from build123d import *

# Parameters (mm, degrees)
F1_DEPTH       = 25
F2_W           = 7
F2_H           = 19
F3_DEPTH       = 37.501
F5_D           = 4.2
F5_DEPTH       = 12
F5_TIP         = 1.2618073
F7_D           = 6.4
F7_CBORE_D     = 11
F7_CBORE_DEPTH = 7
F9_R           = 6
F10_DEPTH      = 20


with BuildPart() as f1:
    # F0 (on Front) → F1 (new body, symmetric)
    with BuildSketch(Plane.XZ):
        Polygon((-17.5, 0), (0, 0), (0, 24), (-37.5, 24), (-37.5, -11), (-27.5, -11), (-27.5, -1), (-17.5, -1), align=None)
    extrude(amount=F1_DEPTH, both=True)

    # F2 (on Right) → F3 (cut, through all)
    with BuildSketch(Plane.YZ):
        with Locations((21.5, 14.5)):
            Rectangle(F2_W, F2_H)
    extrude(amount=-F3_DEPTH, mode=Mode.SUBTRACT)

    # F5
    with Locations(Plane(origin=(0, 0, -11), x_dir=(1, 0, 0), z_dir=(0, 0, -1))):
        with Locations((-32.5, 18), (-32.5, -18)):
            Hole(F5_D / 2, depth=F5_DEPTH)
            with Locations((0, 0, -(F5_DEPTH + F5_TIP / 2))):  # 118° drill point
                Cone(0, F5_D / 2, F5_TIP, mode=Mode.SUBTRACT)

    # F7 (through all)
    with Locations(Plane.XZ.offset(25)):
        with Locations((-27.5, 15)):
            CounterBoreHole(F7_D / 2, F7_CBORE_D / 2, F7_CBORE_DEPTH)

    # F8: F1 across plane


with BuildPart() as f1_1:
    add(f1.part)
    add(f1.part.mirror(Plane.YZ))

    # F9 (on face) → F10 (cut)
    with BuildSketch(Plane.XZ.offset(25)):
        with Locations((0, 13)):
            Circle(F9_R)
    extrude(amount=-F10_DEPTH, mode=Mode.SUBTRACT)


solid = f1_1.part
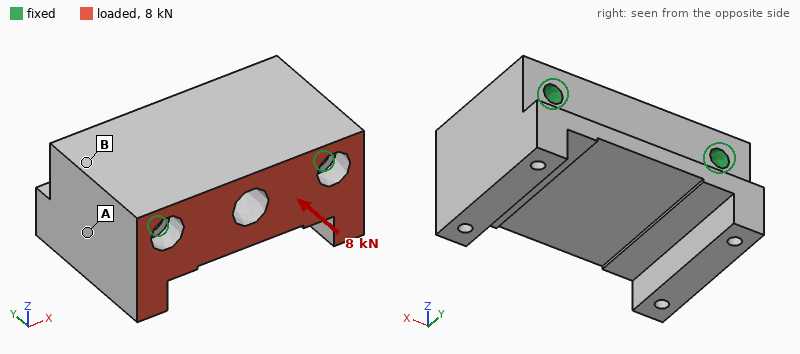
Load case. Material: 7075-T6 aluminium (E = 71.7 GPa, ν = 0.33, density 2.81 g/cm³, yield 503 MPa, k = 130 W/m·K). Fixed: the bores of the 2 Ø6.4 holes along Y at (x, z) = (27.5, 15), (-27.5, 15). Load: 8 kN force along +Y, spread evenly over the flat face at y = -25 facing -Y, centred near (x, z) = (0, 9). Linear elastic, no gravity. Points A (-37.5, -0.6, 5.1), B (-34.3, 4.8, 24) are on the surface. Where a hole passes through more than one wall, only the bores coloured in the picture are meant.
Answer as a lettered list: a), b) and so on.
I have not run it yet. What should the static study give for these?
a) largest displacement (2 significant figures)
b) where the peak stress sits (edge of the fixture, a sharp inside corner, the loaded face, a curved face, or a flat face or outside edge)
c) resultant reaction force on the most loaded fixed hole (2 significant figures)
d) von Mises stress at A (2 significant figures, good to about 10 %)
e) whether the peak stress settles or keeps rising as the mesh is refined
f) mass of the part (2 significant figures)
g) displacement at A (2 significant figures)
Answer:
a) 4.7 µm
b) edge of the fixture
c) 4.0 kN
d) 3.8 MPa
e) keeps rising
f) 240 g
g) 1.1 µm
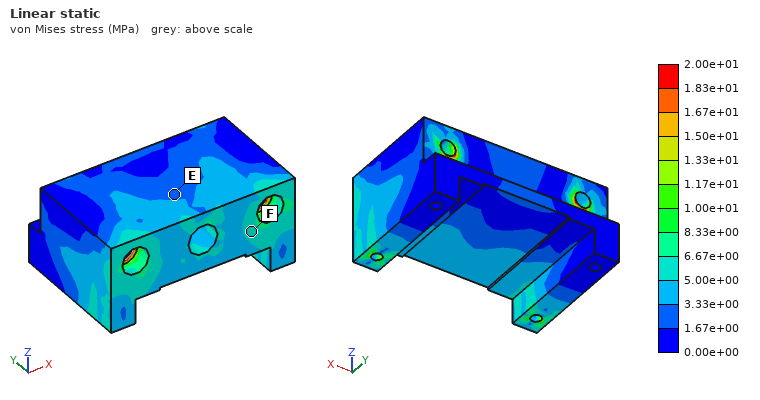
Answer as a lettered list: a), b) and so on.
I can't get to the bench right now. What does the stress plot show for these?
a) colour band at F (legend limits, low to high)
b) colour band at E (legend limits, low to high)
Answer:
a) 5.00e+00 to 6.67e+00 MPa
b) 1.67e+00 to 3.33e+00 MPa
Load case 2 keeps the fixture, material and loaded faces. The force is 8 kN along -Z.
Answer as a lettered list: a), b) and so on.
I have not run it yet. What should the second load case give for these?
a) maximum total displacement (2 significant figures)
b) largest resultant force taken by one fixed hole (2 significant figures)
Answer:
a) 15 µm
b) 4.0 kN
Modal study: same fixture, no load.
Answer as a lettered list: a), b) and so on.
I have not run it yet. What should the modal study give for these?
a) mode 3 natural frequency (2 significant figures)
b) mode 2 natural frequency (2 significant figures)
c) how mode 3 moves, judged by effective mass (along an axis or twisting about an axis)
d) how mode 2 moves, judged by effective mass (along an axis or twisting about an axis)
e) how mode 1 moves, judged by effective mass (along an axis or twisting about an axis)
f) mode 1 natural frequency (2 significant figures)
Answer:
a) 20 kHz
b) 19 kHz
c) along X
d) along Y
e) along Z
f) 16 kHz
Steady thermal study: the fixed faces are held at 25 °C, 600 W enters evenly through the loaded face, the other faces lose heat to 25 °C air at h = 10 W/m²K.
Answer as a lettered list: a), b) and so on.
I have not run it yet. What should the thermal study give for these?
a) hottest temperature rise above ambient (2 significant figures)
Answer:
a) 66 K
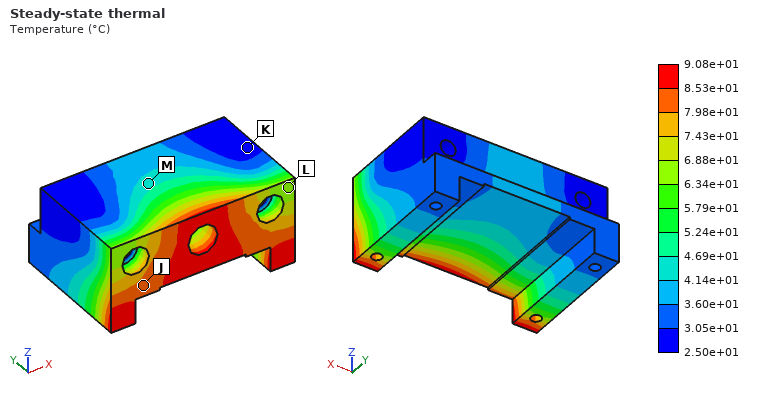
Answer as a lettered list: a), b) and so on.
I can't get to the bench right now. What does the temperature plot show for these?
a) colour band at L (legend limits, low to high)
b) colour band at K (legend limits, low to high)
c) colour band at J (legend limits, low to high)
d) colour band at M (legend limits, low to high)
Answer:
a) 6.34e+01 to 6.88e+01 °C
b) 2.50e+01 to 3.05e+01 °C
c) 7.98e+01 to 8.53e+01 °C
d) 4.14e+01 to 4.69e+01 °C
